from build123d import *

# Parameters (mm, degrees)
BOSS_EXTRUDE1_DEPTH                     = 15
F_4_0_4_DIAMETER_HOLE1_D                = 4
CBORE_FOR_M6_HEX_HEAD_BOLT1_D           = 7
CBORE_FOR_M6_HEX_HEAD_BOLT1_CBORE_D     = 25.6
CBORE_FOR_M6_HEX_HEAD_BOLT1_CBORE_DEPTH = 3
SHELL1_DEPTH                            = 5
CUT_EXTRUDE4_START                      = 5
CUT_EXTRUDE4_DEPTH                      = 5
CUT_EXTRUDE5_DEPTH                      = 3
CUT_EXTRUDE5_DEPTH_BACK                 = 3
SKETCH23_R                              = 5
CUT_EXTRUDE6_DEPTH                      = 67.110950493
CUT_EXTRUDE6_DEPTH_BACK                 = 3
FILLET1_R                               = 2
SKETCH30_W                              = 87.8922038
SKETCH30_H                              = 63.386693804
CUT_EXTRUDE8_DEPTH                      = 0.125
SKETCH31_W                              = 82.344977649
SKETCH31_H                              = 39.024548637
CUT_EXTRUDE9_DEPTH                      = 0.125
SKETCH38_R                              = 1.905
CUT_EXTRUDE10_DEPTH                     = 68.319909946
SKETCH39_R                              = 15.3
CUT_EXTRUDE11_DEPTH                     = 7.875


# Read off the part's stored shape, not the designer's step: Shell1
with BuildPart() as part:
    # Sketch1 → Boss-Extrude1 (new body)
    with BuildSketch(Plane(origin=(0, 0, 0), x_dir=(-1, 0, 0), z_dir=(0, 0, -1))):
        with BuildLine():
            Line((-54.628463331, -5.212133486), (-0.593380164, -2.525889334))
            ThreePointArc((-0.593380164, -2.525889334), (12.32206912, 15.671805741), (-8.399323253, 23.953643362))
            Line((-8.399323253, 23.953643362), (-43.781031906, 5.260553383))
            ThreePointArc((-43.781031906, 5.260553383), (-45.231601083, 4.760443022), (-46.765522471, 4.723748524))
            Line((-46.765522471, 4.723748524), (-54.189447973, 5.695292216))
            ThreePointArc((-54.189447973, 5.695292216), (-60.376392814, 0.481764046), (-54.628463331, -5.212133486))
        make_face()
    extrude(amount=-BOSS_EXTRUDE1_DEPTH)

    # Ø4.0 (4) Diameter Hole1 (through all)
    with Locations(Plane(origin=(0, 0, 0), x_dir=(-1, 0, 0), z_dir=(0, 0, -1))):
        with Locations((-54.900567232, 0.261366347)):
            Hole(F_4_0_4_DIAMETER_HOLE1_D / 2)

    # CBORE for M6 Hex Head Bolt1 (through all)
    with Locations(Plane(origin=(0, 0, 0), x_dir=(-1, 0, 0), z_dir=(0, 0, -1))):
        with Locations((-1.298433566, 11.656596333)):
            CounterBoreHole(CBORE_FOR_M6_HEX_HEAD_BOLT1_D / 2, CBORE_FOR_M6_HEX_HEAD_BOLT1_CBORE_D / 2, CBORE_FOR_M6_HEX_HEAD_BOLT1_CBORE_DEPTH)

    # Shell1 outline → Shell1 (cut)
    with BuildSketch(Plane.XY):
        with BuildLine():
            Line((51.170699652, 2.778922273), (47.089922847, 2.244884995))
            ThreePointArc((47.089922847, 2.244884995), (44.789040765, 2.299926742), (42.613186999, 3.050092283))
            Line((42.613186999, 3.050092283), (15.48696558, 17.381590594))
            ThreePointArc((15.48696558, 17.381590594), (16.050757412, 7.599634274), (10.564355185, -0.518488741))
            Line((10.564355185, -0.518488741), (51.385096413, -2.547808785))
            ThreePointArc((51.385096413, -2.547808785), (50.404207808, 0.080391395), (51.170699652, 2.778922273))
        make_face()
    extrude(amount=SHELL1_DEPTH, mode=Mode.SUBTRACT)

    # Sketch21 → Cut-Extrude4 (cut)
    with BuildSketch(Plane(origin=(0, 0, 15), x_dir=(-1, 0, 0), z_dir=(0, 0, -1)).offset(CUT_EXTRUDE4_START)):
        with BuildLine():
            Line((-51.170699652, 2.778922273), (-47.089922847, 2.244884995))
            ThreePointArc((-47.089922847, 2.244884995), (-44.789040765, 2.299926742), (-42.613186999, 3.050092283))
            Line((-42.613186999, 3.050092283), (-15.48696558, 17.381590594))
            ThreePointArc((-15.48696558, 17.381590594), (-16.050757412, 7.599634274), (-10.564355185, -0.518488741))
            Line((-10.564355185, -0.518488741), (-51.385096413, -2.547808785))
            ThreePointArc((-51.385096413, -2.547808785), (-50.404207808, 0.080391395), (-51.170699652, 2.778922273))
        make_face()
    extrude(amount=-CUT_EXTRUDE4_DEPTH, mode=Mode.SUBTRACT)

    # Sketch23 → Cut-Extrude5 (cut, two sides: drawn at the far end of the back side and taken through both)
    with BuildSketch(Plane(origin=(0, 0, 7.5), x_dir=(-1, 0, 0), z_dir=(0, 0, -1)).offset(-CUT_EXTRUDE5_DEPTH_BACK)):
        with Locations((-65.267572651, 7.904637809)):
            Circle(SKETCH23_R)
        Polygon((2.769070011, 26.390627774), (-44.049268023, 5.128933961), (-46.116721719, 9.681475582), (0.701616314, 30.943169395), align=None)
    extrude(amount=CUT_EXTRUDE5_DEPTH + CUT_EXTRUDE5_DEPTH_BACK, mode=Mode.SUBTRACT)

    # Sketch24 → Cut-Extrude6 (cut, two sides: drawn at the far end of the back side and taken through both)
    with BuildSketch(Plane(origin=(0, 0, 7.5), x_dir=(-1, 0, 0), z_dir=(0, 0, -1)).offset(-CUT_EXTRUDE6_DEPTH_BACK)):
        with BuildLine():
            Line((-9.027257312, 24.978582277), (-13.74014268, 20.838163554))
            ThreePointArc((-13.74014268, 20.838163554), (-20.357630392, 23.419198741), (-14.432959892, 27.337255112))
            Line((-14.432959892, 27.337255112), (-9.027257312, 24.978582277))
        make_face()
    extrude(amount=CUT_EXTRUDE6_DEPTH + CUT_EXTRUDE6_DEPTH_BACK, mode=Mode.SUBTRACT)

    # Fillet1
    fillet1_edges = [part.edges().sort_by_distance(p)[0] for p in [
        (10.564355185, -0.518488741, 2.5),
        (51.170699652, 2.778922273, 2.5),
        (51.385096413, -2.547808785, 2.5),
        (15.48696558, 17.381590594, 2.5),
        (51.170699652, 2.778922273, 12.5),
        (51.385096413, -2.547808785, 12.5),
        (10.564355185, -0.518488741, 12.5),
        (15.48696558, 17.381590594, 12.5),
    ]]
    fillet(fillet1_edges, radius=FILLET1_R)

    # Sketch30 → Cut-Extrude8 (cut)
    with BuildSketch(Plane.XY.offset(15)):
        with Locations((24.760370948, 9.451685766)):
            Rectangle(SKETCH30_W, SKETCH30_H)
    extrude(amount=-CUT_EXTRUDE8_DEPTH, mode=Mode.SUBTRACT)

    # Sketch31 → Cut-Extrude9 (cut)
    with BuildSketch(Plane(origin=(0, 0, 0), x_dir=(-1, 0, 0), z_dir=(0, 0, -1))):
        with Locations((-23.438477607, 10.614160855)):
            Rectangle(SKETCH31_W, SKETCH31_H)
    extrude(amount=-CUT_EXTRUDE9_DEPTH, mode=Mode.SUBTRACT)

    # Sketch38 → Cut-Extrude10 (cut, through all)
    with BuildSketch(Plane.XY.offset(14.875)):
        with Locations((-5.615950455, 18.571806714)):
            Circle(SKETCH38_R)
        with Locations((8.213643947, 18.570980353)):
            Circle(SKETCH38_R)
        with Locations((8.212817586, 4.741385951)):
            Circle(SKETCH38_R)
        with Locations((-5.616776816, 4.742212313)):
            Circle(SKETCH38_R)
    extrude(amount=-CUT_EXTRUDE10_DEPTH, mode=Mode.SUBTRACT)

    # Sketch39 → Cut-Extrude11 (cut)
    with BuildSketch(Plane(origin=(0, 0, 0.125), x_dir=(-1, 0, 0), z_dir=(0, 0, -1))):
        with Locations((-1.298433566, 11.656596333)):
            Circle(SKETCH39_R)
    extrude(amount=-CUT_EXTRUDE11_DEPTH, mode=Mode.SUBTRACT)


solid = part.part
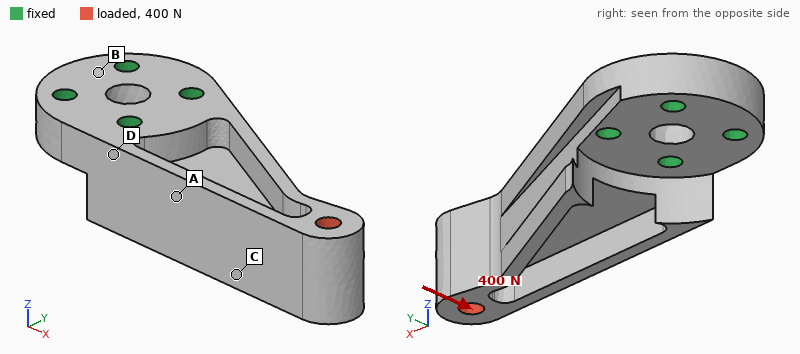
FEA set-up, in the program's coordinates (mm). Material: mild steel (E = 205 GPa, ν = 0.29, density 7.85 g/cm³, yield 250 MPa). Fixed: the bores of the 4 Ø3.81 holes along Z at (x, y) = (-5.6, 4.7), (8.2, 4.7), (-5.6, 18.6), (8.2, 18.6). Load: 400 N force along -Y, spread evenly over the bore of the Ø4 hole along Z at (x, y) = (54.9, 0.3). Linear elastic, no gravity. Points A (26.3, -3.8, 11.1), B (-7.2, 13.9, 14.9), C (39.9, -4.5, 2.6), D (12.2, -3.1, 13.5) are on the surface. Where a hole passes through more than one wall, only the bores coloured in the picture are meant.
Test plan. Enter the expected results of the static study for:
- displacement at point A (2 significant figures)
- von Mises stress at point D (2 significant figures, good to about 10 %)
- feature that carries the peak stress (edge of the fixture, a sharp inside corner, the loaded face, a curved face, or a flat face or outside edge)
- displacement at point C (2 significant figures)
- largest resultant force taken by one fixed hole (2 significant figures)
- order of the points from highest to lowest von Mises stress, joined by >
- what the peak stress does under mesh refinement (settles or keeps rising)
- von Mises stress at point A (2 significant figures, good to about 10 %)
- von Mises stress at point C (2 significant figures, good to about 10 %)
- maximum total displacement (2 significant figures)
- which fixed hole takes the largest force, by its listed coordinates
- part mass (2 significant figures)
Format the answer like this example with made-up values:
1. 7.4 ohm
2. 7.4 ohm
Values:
1. 5.8 µm
2. 36 MPa
3. a sharp inside corner
4. 10.0 µm
5. 1.1 kN
6. D > A > C > B
7. keeps rising
8. 27 MPa
9. 20 MPa
10. 29 µm
11. (8.2, 18.6)
12. 77 g
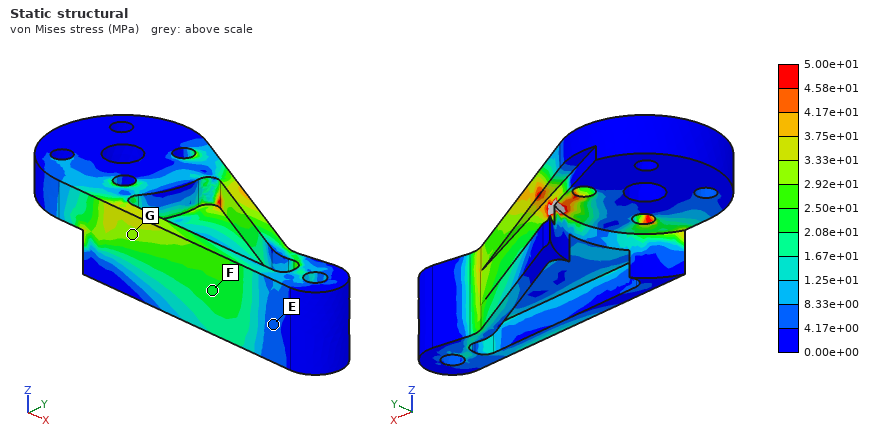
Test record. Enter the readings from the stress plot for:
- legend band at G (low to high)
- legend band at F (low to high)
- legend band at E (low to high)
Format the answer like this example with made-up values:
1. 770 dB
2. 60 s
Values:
1. 2.92e+01 to 3.33e+01 MPa
2. 2.08e+01 to 2.50e+01 MPa
3. 4.17e+00 to 8.33e+00 MPa
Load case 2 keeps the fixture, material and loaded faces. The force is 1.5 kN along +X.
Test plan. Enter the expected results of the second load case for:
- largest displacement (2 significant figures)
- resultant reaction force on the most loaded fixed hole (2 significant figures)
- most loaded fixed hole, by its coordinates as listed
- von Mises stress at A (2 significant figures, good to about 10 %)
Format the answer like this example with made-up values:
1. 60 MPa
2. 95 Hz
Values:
1. 25 µm
2. 1.4 kN
3. (8.2, 4.7)
4. 25 MPa
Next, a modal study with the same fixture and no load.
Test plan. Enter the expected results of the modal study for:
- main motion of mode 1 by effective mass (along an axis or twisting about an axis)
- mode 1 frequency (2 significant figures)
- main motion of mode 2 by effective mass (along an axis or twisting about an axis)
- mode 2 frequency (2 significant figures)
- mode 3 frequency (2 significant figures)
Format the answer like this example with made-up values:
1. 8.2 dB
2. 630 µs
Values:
1. along Z
2. 2200 Hz
3. along Y
4. 5500 Hz
5. 9100 Hz
